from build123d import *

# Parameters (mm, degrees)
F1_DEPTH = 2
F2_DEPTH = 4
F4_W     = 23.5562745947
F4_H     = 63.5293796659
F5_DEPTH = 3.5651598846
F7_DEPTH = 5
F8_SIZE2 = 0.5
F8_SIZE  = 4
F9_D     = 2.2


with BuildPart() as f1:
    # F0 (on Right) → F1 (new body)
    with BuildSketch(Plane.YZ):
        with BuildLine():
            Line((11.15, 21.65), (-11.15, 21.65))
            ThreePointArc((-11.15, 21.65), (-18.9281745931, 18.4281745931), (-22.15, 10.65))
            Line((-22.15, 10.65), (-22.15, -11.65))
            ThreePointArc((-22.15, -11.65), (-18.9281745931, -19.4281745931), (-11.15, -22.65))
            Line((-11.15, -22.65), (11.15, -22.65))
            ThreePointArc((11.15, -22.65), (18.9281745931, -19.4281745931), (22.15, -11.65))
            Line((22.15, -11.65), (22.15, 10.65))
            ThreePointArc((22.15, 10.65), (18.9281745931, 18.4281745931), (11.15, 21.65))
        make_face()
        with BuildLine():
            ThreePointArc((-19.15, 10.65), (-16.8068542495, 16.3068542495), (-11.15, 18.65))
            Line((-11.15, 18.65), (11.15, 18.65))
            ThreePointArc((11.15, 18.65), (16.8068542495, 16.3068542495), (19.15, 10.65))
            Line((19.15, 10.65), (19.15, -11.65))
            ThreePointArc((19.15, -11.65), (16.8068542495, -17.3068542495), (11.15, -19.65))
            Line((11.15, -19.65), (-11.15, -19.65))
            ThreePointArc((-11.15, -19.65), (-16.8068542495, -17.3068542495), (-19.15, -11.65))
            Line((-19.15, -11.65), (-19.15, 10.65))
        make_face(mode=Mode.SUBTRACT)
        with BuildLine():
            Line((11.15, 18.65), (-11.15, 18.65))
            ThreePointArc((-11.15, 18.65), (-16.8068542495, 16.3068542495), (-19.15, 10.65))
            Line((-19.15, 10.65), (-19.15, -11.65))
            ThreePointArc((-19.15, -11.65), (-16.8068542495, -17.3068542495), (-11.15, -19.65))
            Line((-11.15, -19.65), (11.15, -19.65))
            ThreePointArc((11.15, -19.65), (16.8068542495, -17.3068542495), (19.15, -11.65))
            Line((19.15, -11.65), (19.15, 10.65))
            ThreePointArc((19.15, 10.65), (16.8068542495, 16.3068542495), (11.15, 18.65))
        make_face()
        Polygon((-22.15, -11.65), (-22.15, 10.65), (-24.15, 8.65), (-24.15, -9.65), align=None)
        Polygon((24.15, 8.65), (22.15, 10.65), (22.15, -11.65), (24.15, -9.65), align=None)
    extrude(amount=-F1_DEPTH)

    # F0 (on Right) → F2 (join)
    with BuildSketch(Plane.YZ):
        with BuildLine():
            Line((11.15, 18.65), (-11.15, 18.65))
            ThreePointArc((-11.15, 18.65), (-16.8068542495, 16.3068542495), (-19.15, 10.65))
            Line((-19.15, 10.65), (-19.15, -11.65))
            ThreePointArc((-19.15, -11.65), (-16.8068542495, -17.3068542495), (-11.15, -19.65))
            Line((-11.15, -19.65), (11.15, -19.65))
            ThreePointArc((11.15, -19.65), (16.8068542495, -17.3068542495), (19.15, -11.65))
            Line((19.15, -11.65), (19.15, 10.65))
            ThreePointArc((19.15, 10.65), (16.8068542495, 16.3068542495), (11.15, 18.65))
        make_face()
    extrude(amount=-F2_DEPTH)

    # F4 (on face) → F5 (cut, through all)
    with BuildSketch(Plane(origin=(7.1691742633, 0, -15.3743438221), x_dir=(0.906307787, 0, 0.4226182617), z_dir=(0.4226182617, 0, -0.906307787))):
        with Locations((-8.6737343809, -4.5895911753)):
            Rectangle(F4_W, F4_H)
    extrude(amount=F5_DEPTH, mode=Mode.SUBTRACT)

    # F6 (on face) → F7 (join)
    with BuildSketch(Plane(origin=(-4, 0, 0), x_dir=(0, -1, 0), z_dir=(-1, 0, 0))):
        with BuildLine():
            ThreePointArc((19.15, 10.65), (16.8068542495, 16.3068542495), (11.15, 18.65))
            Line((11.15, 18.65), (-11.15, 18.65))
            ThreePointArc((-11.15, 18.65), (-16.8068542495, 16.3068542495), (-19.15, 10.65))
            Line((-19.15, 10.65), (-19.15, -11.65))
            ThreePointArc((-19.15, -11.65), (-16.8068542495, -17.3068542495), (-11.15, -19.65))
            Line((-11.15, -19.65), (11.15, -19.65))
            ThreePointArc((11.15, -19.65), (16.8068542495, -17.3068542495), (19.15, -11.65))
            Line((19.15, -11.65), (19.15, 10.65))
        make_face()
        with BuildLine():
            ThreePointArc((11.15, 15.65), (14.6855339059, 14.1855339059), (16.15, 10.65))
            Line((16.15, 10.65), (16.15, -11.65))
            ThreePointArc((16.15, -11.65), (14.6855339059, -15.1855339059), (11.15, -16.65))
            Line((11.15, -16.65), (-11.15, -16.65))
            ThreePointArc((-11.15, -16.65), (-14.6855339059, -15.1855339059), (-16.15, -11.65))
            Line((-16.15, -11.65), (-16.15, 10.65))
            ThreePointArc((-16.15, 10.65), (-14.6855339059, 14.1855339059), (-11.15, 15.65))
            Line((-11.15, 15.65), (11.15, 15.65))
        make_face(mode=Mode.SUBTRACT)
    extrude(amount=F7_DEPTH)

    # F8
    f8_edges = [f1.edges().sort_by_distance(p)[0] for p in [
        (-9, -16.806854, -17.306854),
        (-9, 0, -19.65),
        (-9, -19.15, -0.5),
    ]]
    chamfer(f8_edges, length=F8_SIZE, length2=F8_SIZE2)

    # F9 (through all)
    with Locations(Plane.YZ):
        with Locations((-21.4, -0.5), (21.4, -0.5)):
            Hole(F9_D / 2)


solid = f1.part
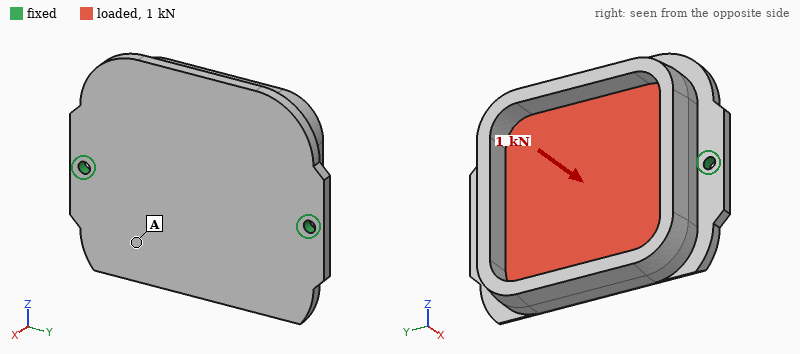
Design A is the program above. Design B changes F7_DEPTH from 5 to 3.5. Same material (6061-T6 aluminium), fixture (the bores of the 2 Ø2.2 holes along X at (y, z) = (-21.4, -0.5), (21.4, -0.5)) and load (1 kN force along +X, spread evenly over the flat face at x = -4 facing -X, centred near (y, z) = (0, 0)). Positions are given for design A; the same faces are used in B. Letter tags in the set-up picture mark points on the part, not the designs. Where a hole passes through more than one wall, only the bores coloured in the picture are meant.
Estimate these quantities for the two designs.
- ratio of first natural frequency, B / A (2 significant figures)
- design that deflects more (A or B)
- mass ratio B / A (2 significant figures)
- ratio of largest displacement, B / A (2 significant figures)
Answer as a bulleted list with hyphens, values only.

- 1.0
- B
- 0.93
- 1.3
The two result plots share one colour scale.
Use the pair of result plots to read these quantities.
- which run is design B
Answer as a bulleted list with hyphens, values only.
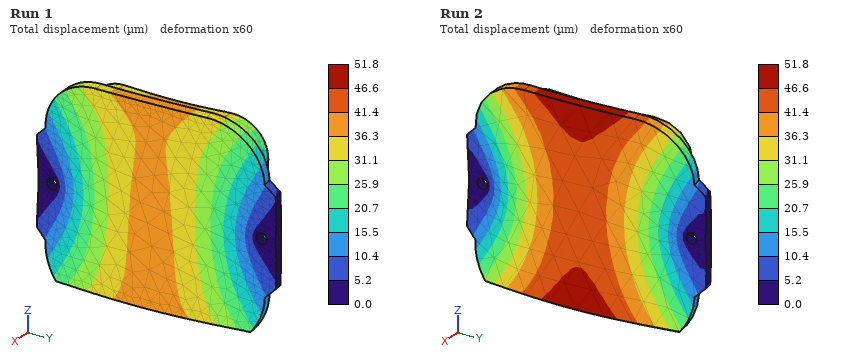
- Run 2
